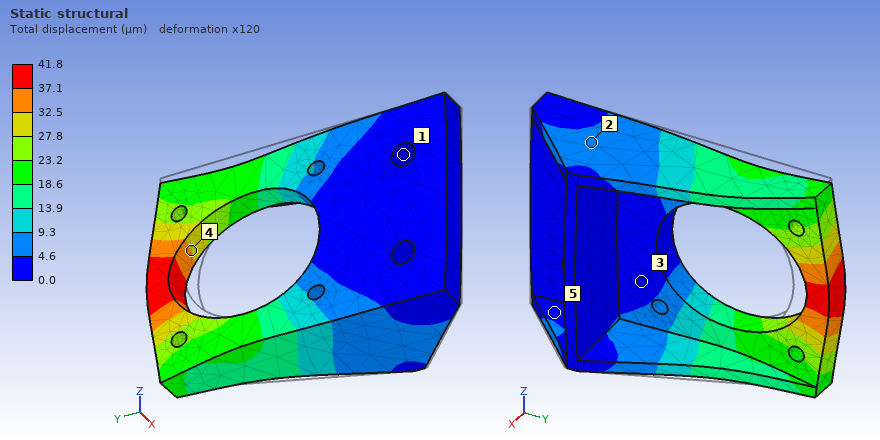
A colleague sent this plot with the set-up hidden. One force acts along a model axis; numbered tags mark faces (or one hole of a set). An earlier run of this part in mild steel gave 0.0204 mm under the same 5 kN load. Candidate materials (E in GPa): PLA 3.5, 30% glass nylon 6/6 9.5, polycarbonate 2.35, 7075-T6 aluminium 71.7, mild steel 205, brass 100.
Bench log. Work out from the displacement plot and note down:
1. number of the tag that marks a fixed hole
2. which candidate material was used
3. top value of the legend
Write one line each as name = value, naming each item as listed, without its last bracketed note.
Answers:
number of the tag that marks a fixed hole = 1
which candidate material was used = brass
top value of the legend = 41.8 µm
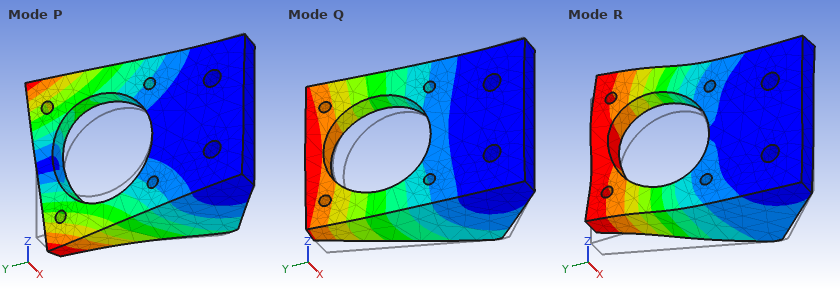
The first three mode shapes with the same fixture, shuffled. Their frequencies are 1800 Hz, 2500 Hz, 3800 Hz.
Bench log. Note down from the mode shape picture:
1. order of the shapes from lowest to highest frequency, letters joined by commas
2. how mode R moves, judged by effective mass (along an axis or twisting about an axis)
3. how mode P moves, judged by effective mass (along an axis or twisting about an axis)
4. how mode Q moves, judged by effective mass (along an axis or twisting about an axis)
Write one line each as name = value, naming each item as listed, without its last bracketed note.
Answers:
order of the shapes from lowest to highest frequency, letters joined by commas = Q, P, R
how mode R moves, judged by effective mass = along Z
how mode P moves, judged by effective mass = twisting about Y
how mode Q moves, judged by effective mass = along X
